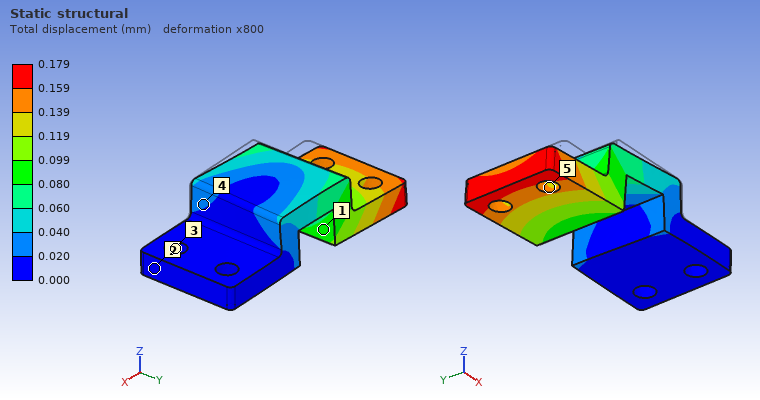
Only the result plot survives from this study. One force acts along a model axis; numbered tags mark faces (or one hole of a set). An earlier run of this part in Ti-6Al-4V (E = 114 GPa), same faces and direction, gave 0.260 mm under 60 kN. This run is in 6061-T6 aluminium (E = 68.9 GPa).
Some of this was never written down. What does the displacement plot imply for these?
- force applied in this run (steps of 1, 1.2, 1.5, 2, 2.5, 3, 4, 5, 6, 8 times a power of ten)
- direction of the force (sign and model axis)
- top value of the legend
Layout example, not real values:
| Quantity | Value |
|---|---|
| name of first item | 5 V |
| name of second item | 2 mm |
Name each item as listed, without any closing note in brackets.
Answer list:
| Quantity | Value |
|---|---|
| force applied in this run | 25 kN |
| direction of the force | +Y |
| top value of the legend | 0.179 mm |
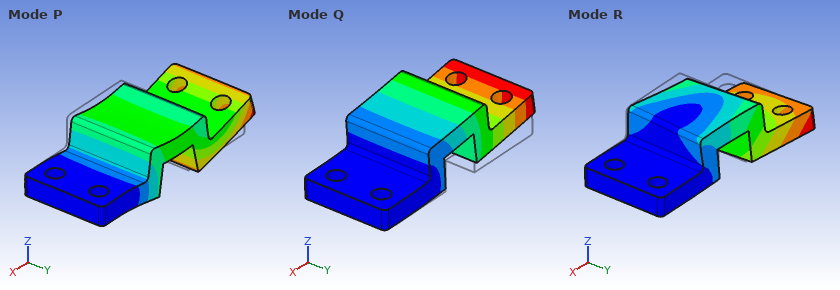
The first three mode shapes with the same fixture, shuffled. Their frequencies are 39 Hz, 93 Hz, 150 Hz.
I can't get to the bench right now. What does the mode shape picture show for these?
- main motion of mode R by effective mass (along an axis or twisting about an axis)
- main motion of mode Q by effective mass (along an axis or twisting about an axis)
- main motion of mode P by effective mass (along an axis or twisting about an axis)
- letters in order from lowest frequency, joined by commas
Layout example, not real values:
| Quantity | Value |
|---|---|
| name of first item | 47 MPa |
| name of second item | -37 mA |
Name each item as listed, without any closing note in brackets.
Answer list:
| Quantity | Value |
|---|---|
| main motion of mode R by effective mass | along Y |
| main motion of mode Q by effective mass | along Z |
| main motion of mode P by effective mass | along X |
| letters in order from lowest frequency, joined by commas | Q, R, P |
